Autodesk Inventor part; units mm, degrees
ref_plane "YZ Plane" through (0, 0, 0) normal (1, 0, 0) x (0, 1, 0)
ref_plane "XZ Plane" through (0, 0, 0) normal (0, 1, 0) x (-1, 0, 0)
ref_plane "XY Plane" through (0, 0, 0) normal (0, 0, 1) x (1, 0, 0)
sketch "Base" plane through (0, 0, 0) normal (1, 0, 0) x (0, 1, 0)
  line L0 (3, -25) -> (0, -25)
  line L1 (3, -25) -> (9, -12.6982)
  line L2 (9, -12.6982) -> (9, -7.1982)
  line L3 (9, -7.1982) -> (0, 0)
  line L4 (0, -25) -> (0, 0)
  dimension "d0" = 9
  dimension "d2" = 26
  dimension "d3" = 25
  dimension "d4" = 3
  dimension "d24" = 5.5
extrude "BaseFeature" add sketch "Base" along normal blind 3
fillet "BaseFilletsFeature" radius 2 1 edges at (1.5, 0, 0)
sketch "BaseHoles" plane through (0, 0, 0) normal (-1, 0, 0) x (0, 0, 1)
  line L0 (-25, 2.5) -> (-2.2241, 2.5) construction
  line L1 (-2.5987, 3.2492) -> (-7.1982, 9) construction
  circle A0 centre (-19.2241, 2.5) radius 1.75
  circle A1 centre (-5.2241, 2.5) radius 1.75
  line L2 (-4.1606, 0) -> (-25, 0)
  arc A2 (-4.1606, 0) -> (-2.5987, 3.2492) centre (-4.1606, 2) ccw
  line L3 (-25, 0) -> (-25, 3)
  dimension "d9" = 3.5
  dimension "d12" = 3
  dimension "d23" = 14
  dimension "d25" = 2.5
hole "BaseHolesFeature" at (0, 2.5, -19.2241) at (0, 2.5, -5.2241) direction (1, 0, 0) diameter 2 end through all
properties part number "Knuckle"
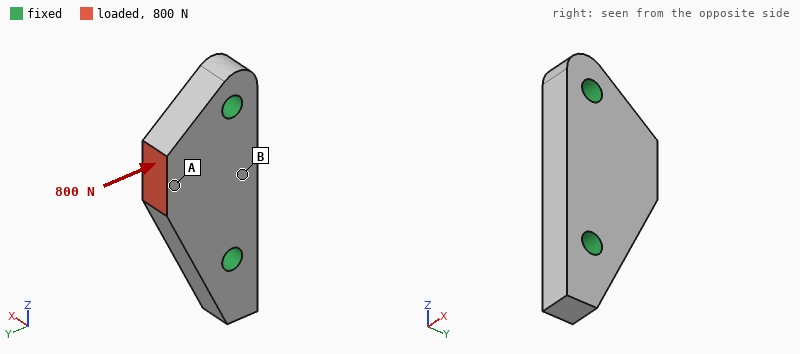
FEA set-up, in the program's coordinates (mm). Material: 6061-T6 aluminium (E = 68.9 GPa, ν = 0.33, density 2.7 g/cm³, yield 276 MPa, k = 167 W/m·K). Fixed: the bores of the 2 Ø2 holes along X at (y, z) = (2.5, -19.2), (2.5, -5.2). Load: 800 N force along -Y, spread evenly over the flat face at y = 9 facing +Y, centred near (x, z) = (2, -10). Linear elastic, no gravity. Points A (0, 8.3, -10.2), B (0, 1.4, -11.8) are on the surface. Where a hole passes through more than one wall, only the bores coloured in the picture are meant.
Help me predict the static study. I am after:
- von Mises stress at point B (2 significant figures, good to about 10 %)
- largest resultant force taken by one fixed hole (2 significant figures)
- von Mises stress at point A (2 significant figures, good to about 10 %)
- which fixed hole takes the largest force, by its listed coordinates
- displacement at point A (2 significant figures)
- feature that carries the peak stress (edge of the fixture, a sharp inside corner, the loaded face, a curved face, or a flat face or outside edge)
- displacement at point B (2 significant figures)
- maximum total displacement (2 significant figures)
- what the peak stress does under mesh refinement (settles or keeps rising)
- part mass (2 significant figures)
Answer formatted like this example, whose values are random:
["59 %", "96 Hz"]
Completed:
["13 MPa", "570 N", "43 MPa", "(2.5, -5.2)", "6.1 µm", "edge of the fixture", "4.1 µm", "6.5 µm", "keeps rising", "1.2 g"]
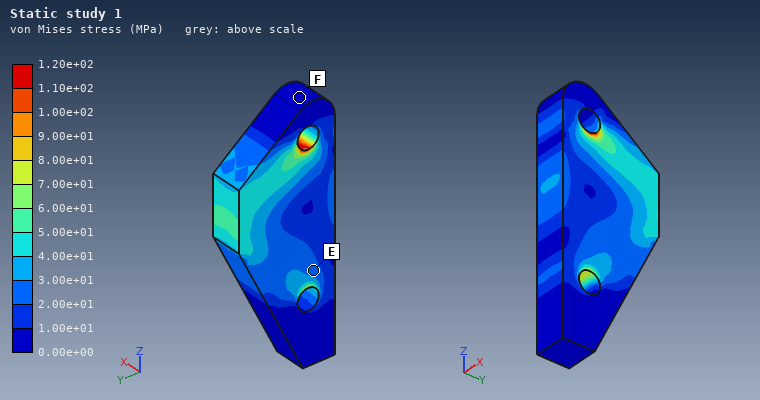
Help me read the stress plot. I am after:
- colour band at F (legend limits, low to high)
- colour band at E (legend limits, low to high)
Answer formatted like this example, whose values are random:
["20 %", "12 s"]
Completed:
["0.00e+00 to 1.00e+01 MPa", "2.00e+01 to 3.00e+01 MPa"]
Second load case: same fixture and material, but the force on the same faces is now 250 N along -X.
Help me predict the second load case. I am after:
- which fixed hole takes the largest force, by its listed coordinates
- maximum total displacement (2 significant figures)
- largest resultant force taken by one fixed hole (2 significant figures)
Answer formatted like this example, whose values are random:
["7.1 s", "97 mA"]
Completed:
["(2.5, -5.2)", "26 µm", "180 N"]
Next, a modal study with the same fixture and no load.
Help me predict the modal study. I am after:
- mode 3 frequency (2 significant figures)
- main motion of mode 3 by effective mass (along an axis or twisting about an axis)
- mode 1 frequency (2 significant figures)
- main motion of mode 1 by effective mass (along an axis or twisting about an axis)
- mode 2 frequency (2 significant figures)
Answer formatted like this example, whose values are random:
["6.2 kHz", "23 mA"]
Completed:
["81 kHz", "along X", "43 kHz", "along X", "74 kHz"]
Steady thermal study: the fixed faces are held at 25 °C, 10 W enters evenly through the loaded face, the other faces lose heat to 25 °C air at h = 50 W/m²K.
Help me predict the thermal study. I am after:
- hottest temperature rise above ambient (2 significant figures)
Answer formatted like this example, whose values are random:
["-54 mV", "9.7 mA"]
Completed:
["18 K"]
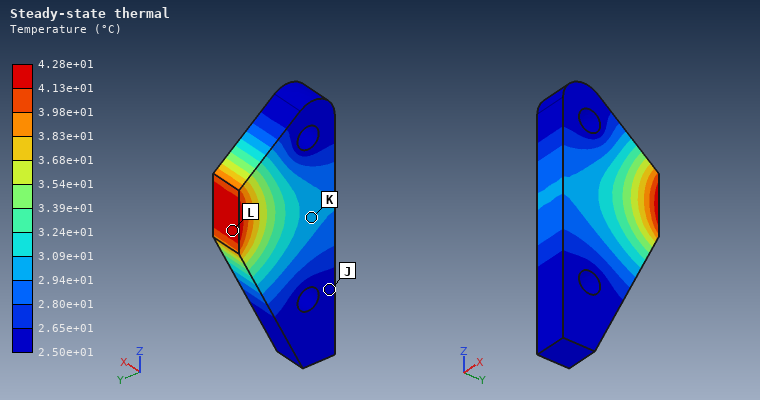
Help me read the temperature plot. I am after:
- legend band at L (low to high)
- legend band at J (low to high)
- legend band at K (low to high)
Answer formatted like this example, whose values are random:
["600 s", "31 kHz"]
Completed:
["4.13e+01 to 4.28e+01 °C", "2.50e+01 to 2.65e+01 °C", "2.94e+01 to 3.09e+01 °C"]
